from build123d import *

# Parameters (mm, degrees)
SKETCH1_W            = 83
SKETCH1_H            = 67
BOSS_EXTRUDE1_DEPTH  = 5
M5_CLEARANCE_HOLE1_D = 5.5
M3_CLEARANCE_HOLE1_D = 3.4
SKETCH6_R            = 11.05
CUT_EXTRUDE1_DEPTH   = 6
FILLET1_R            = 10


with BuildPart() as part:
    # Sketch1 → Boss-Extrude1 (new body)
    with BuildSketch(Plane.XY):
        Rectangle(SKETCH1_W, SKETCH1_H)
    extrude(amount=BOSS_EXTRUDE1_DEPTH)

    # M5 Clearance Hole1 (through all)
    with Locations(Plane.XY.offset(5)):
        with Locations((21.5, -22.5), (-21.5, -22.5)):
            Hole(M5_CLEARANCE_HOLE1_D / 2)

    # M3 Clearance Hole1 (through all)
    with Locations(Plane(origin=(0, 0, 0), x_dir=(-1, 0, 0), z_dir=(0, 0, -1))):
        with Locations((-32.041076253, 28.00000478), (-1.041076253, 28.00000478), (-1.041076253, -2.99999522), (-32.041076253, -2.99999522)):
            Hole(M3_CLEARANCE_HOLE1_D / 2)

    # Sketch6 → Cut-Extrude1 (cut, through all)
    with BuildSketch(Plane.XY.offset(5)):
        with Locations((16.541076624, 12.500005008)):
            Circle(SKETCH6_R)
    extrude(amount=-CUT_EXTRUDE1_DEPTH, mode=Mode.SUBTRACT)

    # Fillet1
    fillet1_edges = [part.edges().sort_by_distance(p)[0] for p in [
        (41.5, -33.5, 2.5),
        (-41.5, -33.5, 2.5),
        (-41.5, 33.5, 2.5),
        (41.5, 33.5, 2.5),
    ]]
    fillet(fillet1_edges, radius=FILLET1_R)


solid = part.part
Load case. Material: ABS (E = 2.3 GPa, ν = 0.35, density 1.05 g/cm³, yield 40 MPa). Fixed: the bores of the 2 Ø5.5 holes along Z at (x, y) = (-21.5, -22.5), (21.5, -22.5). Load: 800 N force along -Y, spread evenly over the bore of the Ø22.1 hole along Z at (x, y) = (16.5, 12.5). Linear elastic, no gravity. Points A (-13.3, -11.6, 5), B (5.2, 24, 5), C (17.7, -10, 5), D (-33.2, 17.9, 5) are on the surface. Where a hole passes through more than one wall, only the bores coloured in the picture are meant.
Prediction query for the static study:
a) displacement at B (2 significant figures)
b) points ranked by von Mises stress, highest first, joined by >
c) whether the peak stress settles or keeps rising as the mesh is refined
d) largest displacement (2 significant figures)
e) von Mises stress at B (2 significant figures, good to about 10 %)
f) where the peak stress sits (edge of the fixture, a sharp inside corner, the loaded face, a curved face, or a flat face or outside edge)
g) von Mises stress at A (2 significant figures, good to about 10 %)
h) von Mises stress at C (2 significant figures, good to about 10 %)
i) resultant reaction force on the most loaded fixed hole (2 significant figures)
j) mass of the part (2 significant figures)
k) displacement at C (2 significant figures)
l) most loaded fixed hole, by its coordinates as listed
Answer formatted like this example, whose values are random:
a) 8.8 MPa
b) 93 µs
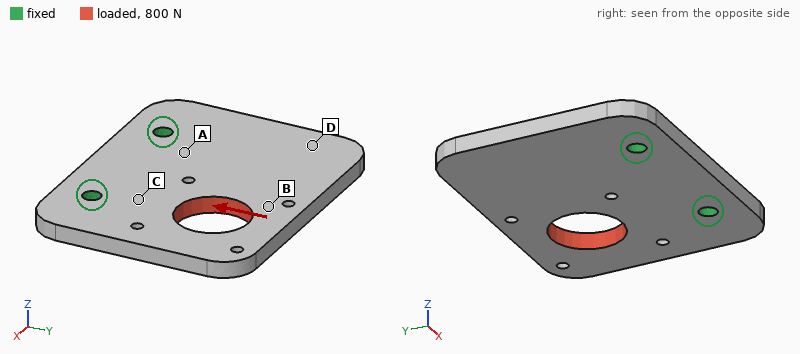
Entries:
a) 0.11 mm
b) C > B > A > D
c) keeps rising
d) 0.16 mm
e) 3.1 MPa
f) edge of the fixture
g) 1.6 MPa
h) 5.0 MPa
i) 690 N
j) 26 g
k) 0.034 mm
l) (21.5, -22.5)
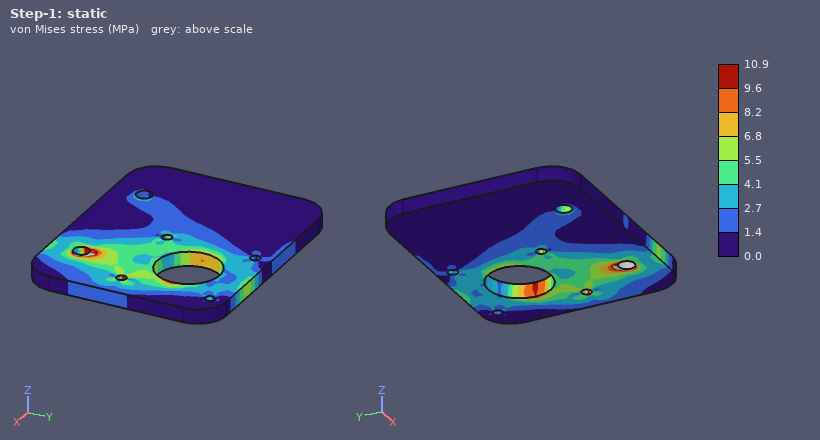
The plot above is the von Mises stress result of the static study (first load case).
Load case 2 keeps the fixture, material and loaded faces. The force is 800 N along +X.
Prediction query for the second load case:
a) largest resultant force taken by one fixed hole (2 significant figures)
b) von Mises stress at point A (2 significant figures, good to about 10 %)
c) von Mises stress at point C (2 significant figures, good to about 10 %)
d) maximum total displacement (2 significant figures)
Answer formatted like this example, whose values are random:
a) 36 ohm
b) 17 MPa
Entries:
a) 730 N
b) 5.6 MPa
c) 7.2 MPa
d) 0.32 mm
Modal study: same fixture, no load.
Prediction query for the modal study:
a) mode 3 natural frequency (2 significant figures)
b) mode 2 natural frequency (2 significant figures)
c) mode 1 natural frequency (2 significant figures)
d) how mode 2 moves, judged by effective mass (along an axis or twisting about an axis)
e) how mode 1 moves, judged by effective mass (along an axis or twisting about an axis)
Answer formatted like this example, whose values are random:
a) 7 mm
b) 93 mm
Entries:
a) 1400 Hz
b) 650 Hz
c) 380 Hz
d) twisting about Y
e) along Z
